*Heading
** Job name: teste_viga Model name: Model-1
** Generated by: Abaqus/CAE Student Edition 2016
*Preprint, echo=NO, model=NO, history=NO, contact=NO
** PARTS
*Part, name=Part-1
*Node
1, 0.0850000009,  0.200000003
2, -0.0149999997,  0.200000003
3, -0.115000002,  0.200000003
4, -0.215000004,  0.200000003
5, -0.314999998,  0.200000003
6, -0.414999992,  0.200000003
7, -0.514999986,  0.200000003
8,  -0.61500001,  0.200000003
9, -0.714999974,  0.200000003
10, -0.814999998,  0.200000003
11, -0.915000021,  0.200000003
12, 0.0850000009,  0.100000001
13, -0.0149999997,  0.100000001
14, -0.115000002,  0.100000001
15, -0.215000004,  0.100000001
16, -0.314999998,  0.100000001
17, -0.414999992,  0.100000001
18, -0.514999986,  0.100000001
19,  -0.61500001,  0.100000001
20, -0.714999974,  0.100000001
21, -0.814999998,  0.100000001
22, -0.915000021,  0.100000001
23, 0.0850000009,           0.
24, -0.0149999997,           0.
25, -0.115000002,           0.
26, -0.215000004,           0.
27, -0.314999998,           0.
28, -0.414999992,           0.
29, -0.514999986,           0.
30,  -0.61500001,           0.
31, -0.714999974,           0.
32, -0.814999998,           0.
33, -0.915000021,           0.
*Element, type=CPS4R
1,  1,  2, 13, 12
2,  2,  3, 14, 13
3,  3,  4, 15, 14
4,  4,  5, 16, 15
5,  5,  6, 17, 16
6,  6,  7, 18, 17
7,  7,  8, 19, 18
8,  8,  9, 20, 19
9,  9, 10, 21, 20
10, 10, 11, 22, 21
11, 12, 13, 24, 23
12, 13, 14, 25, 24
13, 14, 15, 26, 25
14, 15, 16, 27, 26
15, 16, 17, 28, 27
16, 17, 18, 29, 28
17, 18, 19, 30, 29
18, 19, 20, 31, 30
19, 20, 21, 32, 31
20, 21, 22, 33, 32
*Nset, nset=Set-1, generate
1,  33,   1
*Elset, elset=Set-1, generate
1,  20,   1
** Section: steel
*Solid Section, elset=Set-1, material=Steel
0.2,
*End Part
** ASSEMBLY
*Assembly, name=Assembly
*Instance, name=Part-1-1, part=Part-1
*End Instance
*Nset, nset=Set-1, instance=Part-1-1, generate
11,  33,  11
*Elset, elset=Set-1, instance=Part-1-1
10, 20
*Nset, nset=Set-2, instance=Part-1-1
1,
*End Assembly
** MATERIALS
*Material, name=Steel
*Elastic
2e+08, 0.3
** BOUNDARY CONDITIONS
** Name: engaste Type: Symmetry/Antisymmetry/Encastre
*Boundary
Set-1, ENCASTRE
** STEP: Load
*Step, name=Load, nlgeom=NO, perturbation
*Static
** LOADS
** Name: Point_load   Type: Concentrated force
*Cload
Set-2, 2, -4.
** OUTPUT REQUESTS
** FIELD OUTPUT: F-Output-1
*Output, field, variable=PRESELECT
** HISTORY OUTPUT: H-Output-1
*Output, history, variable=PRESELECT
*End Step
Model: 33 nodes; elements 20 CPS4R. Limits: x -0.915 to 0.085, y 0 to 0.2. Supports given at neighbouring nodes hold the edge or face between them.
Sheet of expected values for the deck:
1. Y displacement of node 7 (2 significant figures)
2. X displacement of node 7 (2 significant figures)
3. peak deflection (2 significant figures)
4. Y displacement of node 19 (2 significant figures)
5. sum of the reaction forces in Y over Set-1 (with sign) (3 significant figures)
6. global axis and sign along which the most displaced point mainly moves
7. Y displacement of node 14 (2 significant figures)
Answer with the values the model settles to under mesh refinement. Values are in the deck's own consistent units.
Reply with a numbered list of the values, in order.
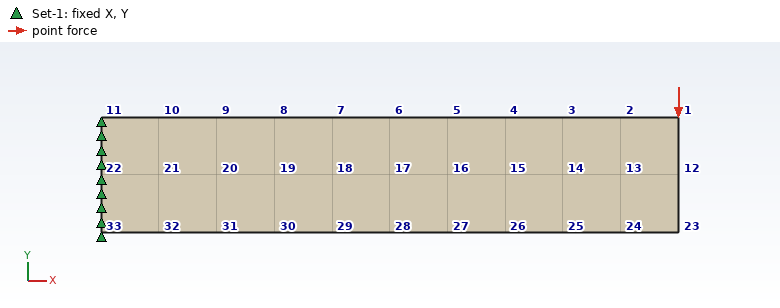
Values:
1. -1.1e-05
2. 4.7e-06
3. 5.1e-05
4. -6.3e-06
5. 4.00
6. -Y
7. -3.5e-05
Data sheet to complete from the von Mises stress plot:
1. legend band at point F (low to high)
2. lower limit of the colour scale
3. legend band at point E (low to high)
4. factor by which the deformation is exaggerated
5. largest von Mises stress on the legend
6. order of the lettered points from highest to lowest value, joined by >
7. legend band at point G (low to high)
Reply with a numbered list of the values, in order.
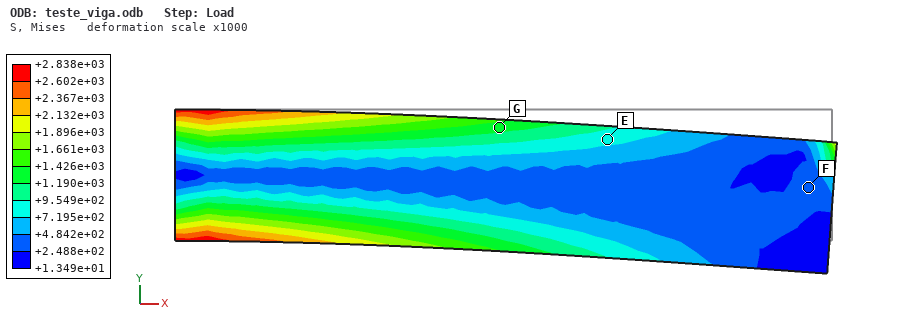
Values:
1. +2.488e+02 to +4.842e+02
2. +1.349e+01
3. +7.195e+02 to +9.549e+02
4. 1000
5. +2.838e+03
6. G > E > F
7. +1.190e+03 to +1.426e+03
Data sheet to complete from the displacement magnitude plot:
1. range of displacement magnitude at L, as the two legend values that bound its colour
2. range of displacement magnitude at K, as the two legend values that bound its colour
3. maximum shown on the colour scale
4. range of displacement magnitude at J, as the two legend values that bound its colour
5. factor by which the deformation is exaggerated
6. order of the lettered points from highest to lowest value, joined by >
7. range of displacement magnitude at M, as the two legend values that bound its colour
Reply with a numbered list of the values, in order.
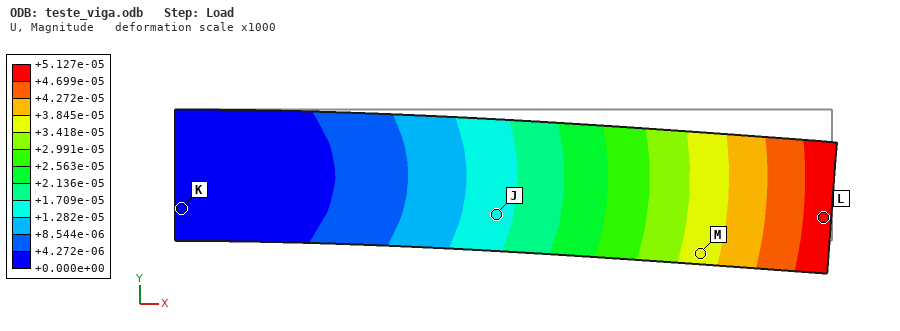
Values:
1. +4.699e-05 to +5.127e-05
2. +0.000e+00 to +4.272e-06
3. +5.127e-05
4. +1.282e-05 to +1.709e-05
5. 1000
6. L > M > J > K
7. +3.418e-05 to +3.845e-05
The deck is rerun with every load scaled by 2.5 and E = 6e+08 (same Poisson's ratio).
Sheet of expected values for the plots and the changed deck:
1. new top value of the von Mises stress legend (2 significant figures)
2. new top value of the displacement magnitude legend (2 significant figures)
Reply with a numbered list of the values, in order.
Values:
1. 7100
2. 4.3e-05
